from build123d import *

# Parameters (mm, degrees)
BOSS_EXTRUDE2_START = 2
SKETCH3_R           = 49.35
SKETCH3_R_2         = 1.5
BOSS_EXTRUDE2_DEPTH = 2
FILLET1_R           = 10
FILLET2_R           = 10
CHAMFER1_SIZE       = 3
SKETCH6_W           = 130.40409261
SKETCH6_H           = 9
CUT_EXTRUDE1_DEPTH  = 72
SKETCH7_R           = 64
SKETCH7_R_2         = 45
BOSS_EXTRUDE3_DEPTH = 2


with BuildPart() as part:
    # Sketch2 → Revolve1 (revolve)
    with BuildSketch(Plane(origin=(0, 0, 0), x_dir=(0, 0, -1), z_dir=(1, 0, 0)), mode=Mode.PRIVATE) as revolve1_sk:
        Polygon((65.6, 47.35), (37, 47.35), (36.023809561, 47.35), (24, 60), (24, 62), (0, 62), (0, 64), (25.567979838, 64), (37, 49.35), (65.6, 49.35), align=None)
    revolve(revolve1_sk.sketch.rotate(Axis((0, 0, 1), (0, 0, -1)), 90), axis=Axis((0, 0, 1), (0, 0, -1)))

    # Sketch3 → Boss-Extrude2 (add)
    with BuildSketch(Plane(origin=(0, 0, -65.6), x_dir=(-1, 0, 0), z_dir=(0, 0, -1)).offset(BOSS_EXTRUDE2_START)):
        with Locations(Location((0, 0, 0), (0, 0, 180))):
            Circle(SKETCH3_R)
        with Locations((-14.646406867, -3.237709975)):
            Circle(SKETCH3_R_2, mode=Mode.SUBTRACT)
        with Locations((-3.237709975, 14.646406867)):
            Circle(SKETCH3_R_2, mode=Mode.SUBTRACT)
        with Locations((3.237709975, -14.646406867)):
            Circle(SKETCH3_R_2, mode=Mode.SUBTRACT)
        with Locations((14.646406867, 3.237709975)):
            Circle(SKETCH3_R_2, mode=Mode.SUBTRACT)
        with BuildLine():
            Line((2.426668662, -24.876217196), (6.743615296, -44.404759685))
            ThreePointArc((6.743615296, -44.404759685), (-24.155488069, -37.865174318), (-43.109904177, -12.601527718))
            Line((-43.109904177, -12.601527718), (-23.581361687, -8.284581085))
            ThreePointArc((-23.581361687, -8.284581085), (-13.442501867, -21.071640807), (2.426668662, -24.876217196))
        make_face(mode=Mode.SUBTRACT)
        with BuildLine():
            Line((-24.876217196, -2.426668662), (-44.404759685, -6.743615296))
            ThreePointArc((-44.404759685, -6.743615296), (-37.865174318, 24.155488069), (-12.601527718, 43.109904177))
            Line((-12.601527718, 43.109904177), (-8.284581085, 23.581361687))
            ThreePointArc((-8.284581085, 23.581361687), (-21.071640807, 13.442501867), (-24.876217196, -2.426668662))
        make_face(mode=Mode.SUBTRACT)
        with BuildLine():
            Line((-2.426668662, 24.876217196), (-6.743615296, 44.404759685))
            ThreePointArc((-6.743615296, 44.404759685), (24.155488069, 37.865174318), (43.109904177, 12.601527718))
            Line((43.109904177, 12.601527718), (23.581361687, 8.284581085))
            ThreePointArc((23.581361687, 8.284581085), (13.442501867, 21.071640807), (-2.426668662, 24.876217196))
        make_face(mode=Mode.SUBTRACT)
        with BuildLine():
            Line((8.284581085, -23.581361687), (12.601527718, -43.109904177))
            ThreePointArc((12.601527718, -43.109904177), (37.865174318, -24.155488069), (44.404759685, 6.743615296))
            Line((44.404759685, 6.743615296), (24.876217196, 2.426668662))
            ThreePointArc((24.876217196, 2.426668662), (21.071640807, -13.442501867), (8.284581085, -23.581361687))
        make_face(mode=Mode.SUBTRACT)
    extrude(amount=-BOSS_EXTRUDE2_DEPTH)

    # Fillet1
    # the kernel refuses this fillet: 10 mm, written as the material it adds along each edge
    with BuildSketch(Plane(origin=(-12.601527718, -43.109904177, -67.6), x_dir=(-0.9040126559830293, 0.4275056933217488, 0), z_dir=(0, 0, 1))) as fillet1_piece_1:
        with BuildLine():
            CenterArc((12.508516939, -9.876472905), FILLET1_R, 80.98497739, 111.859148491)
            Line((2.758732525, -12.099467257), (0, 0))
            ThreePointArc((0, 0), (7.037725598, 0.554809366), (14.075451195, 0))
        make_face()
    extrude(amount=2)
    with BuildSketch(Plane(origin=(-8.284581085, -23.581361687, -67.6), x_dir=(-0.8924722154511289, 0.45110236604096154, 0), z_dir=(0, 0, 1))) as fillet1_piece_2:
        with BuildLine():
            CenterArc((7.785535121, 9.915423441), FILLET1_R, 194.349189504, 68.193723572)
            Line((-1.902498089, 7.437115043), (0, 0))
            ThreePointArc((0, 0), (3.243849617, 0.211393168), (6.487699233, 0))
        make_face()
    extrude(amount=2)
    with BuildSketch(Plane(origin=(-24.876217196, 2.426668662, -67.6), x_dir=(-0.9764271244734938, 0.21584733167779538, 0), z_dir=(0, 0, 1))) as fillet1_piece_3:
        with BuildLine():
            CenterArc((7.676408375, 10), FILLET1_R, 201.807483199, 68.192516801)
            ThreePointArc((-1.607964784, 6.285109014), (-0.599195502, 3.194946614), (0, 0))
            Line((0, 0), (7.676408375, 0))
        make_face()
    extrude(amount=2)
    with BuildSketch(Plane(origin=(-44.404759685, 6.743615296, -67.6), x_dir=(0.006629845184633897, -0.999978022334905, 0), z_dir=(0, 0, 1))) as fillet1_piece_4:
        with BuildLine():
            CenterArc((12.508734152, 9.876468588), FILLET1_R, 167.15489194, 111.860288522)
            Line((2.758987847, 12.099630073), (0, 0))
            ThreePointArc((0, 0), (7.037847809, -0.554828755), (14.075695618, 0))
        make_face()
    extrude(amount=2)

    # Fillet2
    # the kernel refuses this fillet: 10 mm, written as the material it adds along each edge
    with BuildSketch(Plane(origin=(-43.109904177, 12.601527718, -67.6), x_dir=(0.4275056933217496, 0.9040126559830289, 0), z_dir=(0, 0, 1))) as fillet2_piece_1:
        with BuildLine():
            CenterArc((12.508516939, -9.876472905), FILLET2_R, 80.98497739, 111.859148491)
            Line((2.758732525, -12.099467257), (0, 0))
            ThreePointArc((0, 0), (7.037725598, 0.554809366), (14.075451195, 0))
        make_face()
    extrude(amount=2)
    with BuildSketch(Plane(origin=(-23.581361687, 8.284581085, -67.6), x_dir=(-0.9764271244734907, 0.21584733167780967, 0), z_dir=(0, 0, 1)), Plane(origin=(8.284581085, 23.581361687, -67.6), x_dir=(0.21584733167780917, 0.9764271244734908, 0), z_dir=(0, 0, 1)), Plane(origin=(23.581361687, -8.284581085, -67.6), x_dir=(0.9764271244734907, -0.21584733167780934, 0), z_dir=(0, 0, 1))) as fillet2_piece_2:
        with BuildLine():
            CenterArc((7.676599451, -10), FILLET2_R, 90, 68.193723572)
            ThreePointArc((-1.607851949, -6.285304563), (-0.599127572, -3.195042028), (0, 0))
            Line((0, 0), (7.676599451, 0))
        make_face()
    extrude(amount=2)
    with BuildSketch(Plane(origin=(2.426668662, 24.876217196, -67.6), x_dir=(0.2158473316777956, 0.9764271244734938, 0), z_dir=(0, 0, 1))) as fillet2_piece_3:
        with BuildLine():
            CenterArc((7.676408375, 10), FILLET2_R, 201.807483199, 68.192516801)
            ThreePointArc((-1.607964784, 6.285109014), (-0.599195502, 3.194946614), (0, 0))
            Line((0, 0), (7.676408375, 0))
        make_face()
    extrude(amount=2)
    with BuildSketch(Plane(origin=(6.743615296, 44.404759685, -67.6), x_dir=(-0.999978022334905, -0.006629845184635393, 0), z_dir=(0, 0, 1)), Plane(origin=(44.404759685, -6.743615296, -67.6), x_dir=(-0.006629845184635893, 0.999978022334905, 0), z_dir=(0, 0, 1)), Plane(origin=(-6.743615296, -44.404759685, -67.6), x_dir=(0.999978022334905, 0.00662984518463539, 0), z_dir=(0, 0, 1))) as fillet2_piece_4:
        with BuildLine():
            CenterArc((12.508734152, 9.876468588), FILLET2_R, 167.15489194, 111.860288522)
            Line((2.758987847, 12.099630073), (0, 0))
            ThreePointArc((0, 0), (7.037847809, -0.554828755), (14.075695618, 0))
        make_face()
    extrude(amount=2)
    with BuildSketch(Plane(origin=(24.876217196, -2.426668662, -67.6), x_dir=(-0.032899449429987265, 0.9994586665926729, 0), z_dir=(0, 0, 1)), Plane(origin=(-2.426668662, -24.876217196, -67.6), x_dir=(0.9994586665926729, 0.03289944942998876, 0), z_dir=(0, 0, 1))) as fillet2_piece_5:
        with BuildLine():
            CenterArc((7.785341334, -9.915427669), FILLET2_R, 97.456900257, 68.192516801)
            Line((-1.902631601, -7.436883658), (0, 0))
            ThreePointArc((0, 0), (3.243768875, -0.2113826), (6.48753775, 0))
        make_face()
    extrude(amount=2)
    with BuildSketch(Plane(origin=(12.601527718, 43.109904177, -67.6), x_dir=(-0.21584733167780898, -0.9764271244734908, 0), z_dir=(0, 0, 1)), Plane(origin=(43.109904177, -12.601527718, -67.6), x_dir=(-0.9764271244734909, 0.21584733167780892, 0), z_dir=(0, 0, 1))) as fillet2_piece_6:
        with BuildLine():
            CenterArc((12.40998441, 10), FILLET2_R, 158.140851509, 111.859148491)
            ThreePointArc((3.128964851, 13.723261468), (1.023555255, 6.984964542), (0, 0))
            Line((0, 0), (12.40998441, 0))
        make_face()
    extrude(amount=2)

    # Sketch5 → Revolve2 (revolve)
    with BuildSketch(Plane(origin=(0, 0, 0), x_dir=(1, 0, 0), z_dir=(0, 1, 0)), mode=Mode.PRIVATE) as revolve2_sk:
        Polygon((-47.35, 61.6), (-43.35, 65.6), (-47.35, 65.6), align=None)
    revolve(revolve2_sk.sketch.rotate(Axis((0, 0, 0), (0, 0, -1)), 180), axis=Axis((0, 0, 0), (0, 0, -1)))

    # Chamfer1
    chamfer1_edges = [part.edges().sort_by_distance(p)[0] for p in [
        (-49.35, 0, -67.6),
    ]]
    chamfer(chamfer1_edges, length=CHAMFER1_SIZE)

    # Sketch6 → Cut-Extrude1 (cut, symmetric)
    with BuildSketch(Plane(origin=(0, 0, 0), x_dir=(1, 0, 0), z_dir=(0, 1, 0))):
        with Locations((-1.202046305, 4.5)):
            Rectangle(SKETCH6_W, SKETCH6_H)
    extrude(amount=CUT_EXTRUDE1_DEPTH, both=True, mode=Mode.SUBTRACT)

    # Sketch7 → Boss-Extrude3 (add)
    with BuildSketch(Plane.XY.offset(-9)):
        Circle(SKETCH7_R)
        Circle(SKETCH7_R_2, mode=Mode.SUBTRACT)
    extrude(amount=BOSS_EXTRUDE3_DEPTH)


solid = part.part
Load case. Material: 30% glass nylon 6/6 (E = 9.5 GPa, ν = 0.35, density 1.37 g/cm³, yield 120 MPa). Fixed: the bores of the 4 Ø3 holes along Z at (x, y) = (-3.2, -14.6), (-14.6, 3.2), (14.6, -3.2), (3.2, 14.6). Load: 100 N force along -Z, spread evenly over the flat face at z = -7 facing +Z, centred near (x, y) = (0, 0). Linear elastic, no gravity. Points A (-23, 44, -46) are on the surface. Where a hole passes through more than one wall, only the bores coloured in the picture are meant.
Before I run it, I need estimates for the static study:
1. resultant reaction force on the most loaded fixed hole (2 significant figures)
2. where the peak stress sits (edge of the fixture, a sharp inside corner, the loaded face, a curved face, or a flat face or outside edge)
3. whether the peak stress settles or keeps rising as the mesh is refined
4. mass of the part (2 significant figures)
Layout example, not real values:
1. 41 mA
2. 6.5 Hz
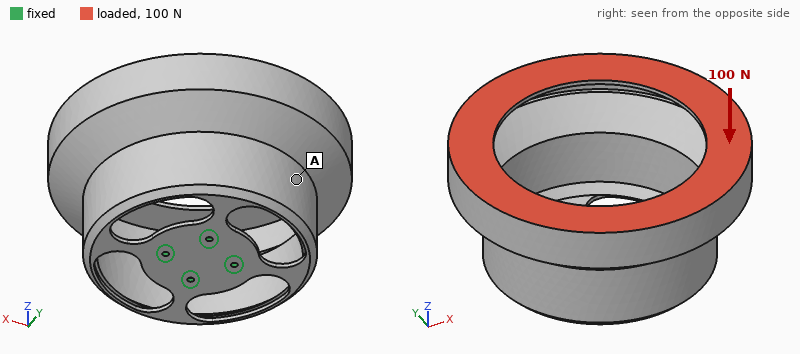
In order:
1. 29 N
2. edge of the fixture
3. keeps rising
4. 98 g
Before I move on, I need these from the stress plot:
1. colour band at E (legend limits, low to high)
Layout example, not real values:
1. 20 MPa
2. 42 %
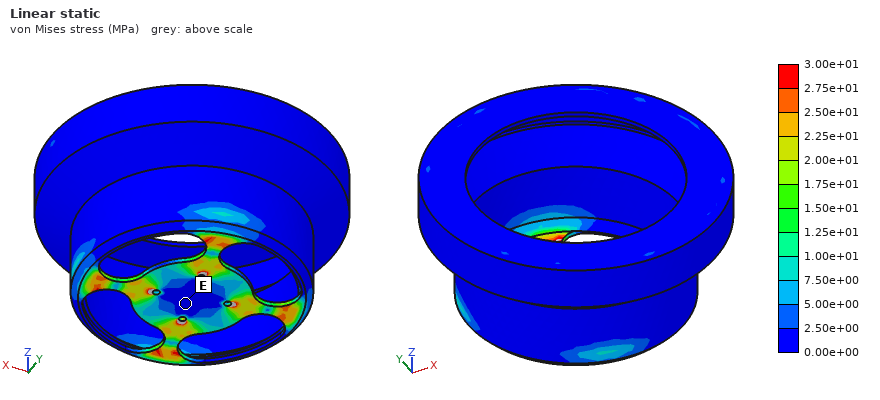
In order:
1. 0.00e+00 to 2.50e+00 MPa
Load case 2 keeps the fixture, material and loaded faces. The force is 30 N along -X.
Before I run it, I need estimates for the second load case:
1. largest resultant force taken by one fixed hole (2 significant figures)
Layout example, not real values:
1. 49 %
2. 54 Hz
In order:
1. 37 N
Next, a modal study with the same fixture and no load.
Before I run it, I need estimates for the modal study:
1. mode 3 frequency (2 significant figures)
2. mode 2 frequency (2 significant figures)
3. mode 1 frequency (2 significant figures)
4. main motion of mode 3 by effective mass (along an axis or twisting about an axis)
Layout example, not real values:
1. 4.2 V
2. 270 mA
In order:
1. 210 Hz
2. 88 Hz
3. 88 Hz
4. along Z
